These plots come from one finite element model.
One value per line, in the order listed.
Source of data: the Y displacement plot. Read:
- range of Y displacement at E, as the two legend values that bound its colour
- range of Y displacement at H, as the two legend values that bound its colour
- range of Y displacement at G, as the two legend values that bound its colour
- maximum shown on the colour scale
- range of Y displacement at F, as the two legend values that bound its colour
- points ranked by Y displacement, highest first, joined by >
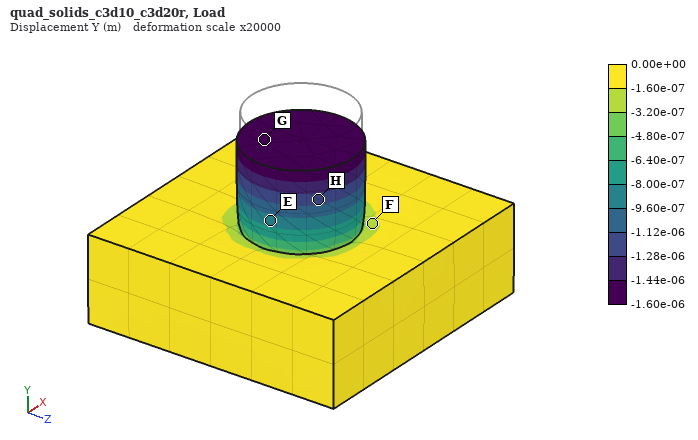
-9.60e-07 to -8.00e-07 m
-1.28e-06 to -1.12e-06 m
-1.60e-06 to -1.44e-06 m
0.00e+00 m
-3.20e-07 to -1.60e-07 m
F > E > H > G
